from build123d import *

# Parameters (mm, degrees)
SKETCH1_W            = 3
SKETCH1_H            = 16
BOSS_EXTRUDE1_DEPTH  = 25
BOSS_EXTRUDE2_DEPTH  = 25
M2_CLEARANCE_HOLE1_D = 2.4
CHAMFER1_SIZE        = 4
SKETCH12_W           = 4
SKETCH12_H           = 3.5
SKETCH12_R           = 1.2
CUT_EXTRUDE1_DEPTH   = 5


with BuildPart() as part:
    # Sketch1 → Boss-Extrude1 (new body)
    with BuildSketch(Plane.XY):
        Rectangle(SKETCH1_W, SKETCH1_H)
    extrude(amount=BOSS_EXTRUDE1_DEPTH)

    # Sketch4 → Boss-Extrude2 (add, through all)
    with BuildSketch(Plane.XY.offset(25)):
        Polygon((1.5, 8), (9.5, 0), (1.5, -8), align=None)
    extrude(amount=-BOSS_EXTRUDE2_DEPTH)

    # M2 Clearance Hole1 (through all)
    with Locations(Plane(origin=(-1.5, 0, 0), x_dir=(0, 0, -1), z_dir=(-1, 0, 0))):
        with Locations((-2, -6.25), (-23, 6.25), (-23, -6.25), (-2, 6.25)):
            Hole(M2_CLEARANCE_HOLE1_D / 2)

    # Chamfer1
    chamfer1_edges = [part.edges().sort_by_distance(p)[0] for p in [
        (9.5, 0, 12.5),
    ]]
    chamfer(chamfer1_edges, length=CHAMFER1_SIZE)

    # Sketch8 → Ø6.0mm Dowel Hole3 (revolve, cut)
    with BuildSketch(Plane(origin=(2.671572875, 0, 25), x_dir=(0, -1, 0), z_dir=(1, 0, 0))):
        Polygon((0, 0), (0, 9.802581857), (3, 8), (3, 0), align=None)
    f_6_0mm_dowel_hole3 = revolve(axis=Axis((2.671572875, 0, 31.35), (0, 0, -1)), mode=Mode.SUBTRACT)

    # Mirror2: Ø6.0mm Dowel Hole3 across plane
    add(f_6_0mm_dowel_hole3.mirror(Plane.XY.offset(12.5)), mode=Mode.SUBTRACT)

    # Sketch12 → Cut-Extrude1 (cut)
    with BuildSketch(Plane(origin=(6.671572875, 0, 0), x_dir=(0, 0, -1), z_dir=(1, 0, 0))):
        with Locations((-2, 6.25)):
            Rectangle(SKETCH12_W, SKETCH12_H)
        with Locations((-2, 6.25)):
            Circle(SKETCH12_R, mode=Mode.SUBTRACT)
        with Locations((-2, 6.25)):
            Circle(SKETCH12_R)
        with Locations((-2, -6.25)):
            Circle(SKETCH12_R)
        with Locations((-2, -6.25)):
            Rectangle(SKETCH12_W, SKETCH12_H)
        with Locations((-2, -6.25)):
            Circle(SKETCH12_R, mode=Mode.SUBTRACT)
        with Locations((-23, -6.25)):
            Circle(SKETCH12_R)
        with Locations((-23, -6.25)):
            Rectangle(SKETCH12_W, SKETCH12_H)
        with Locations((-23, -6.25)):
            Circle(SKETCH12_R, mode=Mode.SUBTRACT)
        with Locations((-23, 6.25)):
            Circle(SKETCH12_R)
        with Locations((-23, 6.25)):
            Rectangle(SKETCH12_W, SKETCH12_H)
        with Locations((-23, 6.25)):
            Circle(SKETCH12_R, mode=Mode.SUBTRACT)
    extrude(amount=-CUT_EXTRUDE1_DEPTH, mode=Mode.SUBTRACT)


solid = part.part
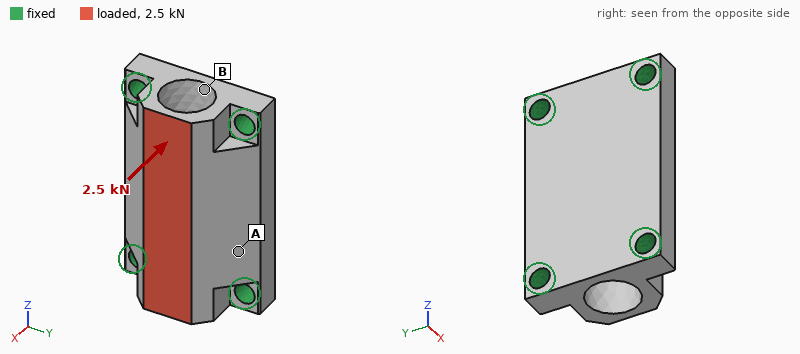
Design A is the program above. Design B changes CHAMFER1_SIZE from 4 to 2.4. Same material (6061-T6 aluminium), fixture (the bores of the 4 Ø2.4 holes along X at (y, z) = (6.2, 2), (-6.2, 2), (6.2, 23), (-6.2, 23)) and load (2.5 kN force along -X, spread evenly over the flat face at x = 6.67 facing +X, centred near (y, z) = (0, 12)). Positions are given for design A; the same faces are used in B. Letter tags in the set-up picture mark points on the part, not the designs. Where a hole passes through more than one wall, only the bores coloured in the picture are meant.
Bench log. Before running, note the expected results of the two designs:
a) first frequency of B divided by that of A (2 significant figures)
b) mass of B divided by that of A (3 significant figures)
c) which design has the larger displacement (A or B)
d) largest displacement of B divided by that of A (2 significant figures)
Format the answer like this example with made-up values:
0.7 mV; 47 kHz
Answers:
1.0; 1.07; A; 0.82
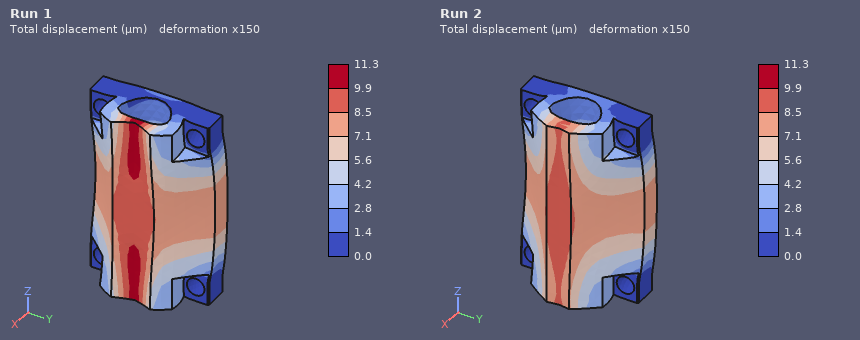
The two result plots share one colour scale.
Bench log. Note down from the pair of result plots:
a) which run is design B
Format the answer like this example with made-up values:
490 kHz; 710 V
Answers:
Run 2
